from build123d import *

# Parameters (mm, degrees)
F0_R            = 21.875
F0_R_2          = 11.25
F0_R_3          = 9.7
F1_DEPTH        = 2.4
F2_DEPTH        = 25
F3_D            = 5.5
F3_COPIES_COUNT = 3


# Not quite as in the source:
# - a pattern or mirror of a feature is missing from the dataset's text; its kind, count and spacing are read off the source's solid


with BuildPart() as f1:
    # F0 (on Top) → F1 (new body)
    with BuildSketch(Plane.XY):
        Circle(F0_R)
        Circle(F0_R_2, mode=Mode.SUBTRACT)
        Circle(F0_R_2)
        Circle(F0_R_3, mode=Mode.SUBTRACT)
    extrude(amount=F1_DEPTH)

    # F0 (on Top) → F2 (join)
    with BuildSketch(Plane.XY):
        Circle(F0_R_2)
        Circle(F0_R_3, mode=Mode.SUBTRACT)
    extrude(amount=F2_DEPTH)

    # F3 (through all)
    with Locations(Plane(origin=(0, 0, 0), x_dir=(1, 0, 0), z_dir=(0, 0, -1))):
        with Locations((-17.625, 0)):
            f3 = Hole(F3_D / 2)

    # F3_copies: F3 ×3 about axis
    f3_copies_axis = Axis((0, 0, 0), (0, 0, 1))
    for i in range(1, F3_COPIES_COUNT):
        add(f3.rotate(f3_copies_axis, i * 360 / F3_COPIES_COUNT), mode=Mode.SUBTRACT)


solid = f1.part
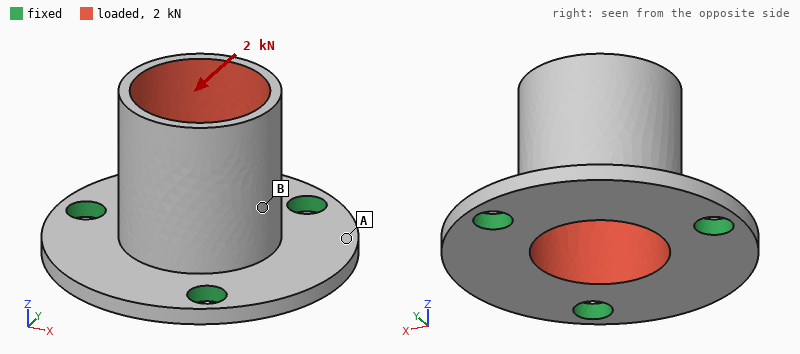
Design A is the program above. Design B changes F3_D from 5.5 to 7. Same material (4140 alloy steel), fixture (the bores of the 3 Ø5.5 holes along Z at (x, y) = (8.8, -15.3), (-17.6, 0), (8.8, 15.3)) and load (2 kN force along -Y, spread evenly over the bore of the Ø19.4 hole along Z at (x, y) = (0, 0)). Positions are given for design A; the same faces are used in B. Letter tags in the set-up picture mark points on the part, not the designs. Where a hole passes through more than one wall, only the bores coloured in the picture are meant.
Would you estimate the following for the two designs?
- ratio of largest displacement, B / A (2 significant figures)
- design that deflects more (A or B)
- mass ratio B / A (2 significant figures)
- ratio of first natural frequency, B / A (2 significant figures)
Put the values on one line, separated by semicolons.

0.83; A; 0.98; 1.1
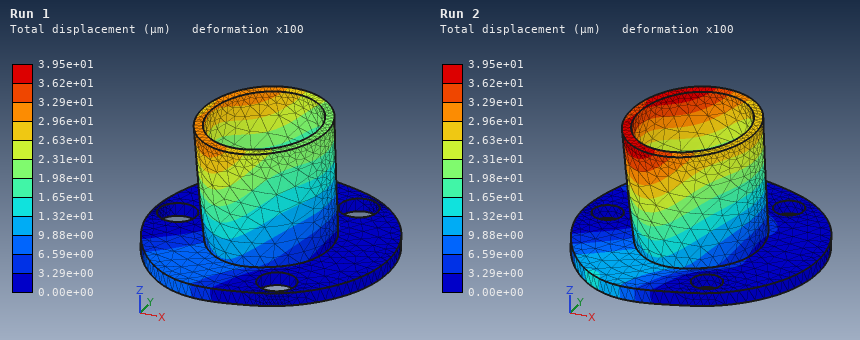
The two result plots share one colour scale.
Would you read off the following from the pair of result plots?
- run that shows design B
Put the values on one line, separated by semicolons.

Run 1
